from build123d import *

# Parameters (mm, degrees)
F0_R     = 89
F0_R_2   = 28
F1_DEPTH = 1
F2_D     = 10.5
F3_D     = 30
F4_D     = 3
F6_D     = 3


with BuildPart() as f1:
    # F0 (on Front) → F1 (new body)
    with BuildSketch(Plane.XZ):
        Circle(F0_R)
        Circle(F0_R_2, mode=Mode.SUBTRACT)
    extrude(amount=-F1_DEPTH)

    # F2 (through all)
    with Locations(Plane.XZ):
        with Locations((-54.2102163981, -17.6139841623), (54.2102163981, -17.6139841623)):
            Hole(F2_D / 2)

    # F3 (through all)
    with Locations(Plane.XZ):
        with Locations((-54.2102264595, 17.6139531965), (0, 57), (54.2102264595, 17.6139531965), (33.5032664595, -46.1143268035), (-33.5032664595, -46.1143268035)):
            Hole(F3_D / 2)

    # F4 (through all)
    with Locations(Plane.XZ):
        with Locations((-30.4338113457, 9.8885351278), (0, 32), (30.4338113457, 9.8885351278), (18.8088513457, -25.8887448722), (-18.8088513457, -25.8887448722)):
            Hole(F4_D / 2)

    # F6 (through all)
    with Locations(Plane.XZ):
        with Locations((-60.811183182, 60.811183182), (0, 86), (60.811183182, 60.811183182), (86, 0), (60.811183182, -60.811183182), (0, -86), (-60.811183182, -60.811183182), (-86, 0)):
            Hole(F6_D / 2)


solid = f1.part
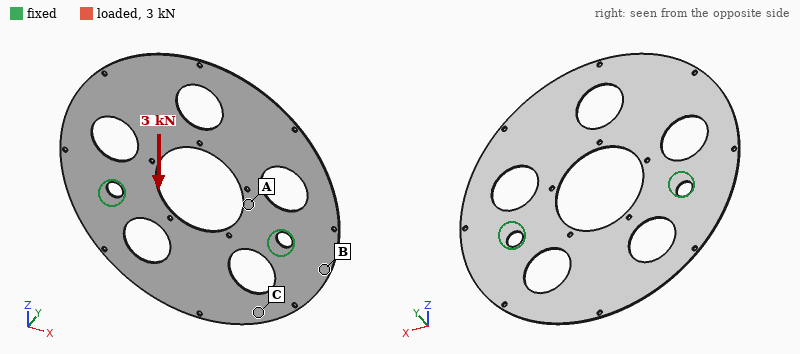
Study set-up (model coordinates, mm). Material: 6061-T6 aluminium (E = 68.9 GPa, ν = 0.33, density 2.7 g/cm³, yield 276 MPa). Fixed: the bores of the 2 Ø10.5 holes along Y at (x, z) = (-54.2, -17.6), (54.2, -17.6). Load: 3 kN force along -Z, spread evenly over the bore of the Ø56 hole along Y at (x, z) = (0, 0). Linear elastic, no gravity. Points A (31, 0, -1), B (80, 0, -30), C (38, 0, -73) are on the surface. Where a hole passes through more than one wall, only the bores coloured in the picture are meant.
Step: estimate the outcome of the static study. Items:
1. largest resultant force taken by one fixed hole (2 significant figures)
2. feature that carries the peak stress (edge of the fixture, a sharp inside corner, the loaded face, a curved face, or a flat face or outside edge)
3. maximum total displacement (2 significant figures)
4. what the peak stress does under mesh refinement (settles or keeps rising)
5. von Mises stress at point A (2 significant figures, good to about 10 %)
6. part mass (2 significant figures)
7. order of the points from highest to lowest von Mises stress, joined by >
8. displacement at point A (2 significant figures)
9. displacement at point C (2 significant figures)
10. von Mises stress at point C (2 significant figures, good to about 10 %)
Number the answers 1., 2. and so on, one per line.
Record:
1. 1.5 kN
2. edge of the fixture
3. 52 µm
4. keeps rising
5. 32 MPa
6. 50 g
7. A > C > B
8. 34 µm
9. 24 µm
10. 19 MPa
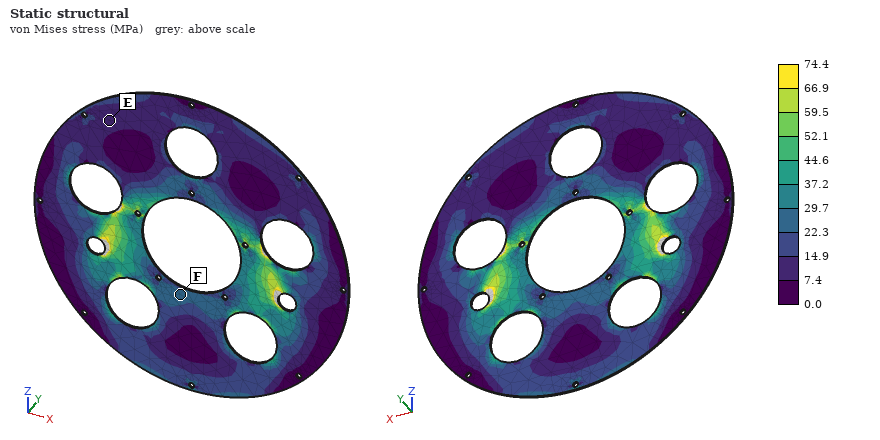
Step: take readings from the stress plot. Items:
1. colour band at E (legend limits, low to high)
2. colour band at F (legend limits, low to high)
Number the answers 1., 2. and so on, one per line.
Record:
1. 7.4 to 14.9 MPa
2. 22.3 to 29.7 MPa
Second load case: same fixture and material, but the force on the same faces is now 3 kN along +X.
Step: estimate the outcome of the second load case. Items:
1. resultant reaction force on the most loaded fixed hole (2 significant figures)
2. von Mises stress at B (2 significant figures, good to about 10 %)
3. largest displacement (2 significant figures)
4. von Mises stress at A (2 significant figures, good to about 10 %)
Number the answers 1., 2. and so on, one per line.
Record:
1. 1.6 kN
2. 16 MPa
3. 92 µm
4. 38 MPa
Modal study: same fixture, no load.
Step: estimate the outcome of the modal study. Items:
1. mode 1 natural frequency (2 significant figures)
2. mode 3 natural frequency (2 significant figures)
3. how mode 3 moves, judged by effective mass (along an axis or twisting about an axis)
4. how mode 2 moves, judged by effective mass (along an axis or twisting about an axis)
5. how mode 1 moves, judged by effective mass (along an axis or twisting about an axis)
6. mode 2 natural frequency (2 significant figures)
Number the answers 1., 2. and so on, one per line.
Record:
1. 73 Hz
2. 180 Hz
3. twisting about Z
4. along Y
5. along Y
6. 160 Hz
